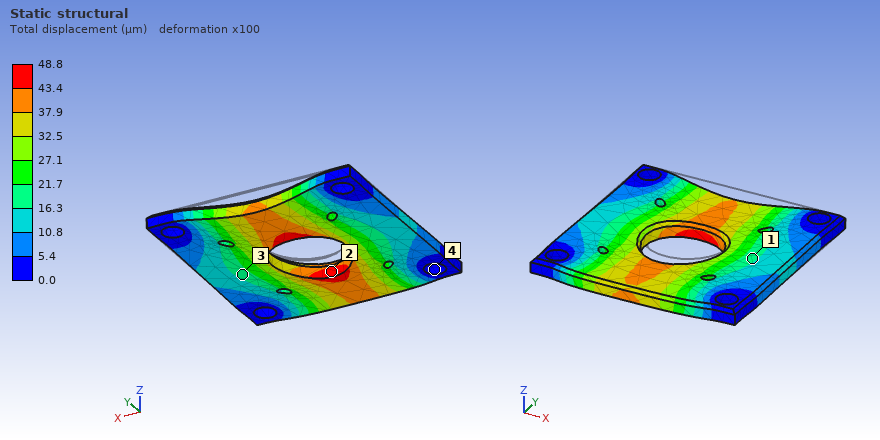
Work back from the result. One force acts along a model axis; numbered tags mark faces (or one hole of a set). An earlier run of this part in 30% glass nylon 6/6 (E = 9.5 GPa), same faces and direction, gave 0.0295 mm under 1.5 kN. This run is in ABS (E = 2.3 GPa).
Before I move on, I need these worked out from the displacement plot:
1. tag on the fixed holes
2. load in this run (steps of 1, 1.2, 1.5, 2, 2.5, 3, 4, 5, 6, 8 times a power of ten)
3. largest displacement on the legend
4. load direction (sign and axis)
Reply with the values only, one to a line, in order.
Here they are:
4
600 N
48.8 µm
-Y
